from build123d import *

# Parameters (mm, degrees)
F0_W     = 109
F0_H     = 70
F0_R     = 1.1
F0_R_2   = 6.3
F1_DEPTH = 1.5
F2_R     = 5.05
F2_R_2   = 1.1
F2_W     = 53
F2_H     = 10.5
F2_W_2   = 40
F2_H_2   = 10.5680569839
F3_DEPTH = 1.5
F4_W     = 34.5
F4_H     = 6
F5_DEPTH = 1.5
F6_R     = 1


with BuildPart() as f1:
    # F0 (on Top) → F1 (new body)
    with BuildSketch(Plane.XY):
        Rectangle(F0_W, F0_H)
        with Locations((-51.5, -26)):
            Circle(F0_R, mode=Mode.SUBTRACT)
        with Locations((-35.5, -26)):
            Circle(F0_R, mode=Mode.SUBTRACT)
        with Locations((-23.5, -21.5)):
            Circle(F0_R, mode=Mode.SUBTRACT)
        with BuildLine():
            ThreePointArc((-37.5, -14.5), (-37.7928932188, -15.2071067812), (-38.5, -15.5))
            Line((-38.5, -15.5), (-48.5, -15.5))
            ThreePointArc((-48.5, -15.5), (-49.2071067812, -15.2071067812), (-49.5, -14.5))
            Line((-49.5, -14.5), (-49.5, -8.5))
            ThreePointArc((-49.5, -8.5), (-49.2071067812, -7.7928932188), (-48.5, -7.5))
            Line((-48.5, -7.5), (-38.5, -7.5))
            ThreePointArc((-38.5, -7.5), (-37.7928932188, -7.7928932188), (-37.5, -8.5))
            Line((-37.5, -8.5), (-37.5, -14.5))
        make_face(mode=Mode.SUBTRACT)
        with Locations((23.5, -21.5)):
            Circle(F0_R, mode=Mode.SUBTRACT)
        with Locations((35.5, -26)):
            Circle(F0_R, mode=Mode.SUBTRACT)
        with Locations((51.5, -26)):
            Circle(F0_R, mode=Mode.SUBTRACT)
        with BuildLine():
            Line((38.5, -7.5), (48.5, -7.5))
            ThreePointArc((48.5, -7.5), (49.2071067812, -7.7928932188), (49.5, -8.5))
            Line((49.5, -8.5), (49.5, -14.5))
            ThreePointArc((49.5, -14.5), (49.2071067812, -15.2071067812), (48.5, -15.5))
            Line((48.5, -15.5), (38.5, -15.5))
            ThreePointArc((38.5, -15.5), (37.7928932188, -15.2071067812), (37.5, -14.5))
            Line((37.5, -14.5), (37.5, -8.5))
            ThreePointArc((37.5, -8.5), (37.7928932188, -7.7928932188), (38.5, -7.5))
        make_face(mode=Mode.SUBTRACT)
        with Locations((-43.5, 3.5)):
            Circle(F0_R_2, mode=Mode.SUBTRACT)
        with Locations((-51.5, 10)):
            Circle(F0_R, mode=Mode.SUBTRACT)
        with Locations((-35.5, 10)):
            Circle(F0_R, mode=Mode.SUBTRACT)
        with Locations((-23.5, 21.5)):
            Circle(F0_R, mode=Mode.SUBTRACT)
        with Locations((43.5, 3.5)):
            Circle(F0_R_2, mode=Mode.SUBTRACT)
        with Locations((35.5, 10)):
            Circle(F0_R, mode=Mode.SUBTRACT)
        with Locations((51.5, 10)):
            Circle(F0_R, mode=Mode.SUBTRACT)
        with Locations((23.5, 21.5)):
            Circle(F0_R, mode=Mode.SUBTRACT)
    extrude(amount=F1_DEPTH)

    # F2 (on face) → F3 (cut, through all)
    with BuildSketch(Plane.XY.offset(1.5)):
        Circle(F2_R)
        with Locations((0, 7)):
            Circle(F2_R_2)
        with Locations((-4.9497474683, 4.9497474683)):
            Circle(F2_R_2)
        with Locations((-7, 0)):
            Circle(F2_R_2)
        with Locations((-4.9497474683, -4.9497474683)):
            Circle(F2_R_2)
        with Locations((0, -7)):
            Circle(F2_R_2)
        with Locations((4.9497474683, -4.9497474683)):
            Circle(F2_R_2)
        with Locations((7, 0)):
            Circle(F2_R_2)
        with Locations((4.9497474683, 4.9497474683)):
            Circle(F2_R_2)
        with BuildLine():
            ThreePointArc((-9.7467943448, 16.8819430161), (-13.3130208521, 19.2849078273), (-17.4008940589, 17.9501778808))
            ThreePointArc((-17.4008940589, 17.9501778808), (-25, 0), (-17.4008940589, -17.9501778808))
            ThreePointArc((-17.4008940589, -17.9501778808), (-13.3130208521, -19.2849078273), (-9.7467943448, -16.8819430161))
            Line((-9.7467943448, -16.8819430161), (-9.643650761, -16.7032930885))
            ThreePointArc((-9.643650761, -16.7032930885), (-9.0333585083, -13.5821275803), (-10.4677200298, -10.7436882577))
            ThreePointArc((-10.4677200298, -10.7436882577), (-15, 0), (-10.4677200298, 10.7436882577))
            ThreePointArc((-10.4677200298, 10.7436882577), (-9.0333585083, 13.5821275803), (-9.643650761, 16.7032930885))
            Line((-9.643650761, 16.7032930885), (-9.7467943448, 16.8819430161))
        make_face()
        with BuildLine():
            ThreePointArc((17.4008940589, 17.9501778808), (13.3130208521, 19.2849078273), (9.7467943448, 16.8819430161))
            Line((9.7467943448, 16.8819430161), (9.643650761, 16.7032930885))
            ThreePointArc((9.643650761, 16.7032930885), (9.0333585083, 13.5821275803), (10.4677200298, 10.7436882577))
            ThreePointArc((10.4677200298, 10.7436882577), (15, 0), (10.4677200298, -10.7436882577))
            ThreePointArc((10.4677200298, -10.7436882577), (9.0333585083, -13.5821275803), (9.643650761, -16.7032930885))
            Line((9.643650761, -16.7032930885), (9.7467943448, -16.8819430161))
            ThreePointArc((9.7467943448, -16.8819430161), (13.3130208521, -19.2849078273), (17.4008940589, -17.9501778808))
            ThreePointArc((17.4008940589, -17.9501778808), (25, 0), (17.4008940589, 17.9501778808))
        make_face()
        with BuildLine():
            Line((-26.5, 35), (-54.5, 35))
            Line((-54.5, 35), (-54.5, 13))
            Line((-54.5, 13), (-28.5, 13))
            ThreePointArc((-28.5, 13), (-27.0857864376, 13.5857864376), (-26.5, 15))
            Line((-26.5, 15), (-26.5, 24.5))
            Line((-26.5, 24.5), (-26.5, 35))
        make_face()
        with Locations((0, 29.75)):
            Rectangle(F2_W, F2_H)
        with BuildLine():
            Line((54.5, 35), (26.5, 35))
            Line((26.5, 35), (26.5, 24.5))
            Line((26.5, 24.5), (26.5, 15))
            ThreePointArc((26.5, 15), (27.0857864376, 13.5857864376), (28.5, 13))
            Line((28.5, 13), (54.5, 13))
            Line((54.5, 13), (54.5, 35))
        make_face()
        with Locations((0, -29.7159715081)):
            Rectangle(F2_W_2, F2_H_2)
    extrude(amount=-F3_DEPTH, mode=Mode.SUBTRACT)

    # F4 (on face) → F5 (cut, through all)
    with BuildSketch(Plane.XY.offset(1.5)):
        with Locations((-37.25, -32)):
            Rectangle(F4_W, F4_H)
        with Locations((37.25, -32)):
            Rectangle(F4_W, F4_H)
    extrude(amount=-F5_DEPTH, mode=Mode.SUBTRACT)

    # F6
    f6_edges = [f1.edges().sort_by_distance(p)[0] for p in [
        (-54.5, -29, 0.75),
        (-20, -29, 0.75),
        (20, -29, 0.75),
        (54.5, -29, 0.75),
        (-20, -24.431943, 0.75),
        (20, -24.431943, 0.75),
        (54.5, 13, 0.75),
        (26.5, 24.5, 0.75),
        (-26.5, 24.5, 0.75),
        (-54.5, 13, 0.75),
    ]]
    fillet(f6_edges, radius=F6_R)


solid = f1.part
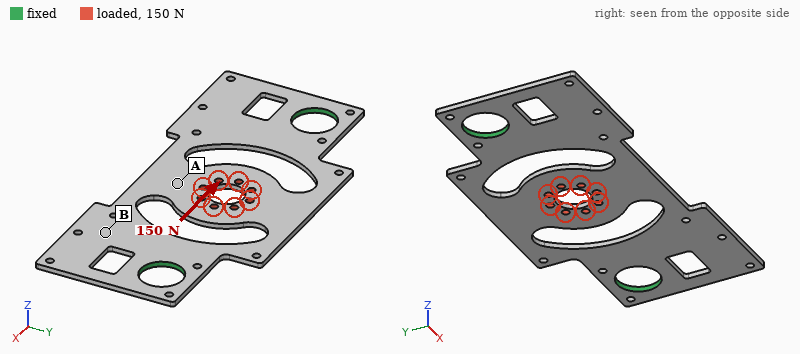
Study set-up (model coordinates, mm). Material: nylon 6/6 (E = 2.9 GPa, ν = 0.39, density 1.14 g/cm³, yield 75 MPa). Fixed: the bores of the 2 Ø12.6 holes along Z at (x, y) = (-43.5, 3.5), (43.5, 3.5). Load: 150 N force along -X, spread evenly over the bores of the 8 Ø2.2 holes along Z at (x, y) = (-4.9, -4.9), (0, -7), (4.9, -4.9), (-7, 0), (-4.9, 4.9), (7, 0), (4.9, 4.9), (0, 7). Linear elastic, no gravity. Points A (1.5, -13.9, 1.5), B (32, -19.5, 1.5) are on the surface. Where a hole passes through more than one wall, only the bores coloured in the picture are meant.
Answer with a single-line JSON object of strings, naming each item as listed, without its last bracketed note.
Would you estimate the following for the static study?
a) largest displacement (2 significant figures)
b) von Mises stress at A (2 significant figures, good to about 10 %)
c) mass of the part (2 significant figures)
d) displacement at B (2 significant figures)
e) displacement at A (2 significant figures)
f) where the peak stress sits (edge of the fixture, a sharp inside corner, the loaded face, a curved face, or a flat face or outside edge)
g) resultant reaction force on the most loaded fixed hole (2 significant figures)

{"largest displacement": "0.24 mm", "von Mises stress at A": "5.5 MPa", "mass of the part": "6.2 g", "displacement at B": "0.080 mm", "displacement at A": "0.17 mm", "where the peak stress sits": "a curved face", "resultant reaction force on the most loaded fixed hole": "76 N"}
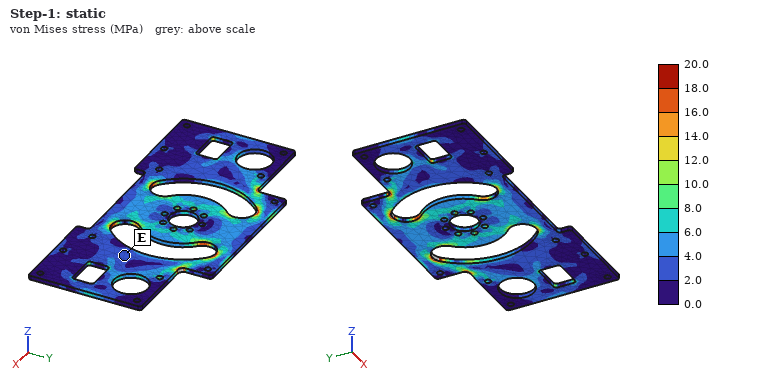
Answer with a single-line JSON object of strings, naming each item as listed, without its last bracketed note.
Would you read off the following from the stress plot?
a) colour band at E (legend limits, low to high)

{"colour band at E": "2.0 to 4.0 MPa"}
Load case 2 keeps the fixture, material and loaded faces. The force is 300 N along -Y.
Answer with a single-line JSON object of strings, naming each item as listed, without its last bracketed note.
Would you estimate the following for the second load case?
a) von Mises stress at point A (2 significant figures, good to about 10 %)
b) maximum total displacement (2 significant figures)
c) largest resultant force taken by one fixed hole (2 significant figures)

{"von Mises stress at point A": "5.5 MPa", "maximum total displacement": "0.55 mm", "largest resultant force taken by one fixed hole": "150 N"}
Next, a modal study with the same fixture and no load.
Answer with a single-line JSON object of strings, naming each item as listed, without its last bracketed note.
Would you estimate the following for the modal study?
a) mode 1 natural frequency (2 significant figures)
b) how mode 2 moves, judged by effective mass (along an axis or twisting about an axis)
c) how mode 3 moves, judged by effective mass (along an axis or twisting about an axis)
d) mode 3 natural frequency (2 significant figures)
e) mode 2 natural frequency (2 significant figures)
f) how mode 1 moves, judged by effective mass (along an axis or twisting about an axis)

{"mode 1 natural frequency": "270 Hz", "how mode 2 moves, judged by effective mass": "twisting about X", "how mode 3 moves, judged by effective mass": "twisting about Y", "mode 3 natural frequency": "440 Hz", "mode 2 natural frequency": "310 Hz", "how mode 1 moves, judged by effective mass": "along Z"}
